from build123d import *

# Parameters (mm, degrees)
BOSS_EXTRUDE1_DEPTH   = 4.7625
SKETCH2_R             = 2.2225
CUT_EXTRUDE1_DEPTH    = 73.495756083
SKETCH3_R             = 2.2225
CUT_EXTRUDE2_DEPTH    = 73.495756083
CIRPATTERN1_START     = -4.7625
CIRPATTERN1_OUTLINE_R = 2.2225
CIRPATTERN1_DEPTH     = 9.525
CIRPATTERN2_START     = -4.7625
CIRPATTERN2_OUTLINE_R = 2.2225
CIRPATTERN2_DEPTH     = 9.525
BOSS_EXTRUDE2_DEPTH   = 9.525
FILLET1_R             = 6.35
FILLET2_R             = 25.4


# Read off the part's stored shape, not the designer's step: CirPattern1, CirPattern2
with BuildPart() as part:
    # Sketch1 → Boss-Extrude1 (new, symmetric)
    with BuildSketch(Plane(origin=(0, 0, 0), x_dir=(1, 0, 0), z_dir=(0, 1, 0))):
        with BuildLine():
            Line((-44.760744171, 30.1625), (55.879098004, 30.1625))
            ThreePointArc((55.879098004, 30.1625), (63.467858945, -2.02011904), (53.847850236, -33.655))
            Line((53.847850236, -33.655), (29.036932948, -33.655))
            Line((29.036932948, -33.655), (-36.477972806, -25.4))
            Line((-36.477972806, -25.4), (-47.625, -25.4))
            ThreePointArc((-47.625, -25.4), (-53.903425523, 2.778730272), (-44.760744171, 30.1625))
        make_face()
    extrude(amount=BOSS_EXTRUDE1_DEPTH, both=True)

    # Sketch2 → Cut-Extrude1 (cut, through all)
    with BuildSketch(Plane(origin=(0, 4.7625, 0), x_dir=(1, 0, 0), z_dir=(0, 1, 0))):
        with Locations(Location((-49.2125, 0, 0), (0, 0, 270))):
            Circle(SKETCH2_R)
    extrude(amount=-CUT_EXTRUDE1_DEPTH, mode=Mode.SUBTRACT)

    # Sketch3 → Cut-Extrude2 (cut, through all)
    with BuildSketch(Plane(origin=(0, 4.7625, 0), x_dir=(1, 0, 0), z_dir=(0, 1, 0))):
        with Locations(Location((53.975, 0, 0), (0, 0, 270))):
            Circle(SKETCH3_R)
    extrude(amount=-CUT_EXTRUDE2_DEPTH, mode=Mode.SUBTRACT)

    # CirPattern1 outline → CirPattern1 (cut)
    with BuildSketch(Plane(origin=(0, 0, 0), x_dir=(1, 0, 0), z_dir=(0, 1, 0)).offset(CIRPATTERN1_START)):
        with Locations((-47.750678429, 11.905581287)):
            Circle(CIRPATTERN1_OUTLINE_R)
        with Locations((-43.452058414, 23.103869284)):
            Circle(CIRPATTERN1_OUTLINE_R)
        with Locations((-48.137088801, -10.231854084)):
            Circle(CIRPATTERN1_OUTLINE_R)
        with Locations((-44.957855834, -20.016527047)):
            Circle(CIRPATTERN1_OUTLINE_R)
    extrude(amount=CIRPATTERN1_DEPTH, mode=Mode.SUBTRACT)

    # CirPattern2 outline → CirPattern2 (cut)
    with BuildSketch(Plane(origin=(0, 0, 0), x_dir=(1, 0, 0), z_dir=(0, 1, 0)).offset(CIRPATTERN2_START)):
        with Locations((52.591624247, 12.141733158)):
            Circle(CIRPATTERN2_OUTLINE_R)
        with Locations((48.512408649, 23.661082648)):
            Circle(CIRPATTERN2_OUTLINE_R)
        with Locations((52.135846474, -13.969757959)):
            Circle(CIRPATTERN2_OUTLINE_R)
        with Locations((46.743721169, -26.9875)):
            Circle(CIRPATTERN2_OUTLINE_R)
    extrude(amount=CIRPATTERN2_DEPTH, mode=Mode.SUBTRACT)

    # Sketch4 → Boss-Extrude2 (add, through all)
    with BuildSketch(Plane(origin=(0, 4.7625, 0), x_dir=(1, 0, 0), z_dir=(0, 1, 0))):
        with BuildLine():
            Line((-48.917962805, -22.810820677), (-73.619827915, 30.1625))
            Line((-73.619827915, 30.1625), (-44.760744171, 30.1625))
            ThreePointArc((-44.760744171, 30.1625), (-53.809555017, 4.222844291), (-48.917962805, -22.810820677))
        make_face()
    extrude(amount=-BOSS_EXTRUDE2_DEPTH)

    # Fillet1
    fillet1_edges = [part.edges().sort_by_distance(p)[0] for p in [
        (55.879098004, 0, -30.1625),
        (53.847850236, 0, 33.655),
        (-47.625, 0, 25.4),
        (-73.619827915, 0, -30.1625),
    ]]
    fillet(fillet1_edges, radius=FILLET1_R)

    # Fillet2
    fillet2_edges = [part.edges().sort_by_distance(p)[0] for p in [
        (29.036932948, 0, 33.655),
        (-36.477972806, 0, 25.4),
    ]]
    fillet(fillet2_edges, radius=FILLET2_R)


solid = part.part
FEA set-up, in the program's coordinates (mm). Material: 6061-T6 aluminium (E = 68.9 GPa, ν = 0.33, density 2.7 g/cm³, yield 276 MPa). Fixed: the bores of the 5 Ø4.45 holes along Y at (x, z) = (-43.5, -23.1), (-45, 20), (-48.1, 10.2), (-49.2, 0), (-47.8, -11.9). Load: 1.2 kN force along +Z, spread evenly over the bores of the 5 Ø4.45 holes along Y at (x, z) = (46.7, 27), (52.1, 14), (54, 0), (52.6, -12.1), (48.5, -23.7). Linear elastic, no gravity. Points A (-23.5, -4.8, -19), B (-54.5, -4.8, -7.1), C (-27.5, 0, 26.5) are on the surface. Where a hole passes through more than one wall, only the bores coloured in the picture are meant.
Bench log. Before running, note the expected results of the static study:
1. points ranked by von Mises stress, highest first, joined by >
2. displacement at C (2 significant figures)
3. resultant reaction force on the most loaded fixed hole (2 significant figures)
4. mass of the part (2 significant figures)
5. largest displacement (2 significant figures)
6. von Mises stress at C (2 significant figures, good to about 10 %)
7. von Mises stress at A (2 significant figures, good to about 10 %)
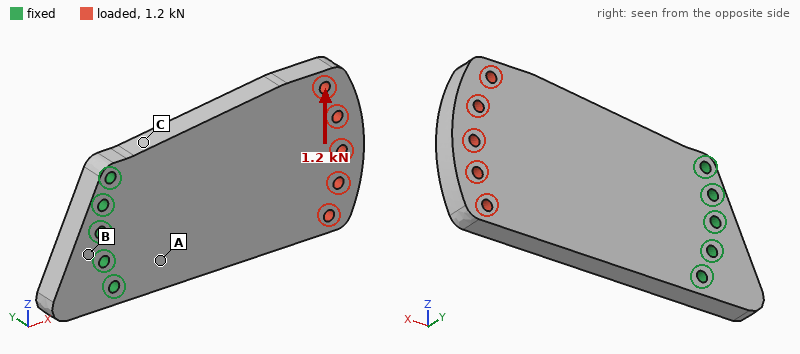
C > A > B
7.8 µm
2.4 kN
180 g
50 µm
18 MPa
12 MPa
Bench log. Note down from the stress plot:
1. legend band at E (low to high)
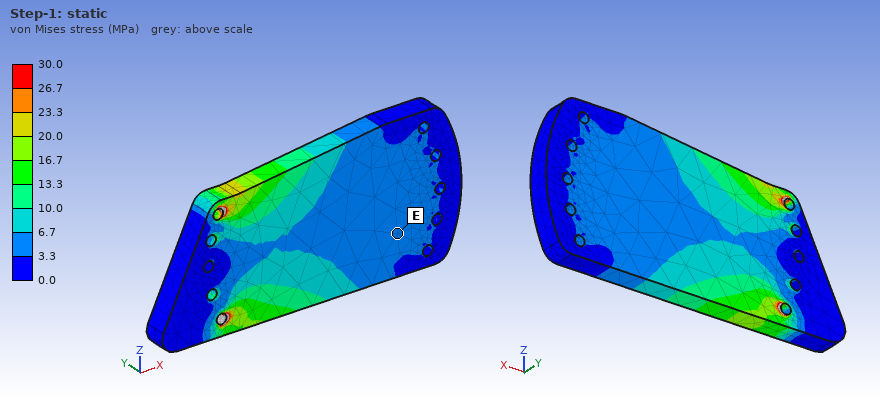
3.3 to 6.7 MPa
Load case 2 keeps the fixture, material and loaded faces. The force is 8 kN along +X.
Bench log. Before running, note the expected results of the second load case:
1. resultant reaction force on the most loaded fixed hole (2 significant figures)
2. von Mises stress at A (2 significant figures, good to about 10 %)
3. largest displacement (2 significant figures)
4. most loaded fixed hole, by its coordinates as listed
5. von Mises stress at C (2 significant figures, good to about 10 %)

2.4 kN
12 MPa
24 µm
(-45, 20)
19 MPa
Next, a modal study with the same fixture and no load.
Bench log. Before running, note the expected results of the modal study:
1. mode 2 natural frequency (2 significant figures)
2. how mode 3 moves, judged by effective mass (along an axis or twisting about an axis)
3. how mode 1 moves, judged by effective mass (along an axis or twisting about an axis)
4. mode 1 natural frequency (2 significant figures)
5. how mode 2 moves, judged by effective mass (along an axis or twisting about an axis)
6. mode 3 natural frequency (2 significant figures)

2400 Hz
along Z
along Y
670 Hz
twisting about X
3300 Hz
